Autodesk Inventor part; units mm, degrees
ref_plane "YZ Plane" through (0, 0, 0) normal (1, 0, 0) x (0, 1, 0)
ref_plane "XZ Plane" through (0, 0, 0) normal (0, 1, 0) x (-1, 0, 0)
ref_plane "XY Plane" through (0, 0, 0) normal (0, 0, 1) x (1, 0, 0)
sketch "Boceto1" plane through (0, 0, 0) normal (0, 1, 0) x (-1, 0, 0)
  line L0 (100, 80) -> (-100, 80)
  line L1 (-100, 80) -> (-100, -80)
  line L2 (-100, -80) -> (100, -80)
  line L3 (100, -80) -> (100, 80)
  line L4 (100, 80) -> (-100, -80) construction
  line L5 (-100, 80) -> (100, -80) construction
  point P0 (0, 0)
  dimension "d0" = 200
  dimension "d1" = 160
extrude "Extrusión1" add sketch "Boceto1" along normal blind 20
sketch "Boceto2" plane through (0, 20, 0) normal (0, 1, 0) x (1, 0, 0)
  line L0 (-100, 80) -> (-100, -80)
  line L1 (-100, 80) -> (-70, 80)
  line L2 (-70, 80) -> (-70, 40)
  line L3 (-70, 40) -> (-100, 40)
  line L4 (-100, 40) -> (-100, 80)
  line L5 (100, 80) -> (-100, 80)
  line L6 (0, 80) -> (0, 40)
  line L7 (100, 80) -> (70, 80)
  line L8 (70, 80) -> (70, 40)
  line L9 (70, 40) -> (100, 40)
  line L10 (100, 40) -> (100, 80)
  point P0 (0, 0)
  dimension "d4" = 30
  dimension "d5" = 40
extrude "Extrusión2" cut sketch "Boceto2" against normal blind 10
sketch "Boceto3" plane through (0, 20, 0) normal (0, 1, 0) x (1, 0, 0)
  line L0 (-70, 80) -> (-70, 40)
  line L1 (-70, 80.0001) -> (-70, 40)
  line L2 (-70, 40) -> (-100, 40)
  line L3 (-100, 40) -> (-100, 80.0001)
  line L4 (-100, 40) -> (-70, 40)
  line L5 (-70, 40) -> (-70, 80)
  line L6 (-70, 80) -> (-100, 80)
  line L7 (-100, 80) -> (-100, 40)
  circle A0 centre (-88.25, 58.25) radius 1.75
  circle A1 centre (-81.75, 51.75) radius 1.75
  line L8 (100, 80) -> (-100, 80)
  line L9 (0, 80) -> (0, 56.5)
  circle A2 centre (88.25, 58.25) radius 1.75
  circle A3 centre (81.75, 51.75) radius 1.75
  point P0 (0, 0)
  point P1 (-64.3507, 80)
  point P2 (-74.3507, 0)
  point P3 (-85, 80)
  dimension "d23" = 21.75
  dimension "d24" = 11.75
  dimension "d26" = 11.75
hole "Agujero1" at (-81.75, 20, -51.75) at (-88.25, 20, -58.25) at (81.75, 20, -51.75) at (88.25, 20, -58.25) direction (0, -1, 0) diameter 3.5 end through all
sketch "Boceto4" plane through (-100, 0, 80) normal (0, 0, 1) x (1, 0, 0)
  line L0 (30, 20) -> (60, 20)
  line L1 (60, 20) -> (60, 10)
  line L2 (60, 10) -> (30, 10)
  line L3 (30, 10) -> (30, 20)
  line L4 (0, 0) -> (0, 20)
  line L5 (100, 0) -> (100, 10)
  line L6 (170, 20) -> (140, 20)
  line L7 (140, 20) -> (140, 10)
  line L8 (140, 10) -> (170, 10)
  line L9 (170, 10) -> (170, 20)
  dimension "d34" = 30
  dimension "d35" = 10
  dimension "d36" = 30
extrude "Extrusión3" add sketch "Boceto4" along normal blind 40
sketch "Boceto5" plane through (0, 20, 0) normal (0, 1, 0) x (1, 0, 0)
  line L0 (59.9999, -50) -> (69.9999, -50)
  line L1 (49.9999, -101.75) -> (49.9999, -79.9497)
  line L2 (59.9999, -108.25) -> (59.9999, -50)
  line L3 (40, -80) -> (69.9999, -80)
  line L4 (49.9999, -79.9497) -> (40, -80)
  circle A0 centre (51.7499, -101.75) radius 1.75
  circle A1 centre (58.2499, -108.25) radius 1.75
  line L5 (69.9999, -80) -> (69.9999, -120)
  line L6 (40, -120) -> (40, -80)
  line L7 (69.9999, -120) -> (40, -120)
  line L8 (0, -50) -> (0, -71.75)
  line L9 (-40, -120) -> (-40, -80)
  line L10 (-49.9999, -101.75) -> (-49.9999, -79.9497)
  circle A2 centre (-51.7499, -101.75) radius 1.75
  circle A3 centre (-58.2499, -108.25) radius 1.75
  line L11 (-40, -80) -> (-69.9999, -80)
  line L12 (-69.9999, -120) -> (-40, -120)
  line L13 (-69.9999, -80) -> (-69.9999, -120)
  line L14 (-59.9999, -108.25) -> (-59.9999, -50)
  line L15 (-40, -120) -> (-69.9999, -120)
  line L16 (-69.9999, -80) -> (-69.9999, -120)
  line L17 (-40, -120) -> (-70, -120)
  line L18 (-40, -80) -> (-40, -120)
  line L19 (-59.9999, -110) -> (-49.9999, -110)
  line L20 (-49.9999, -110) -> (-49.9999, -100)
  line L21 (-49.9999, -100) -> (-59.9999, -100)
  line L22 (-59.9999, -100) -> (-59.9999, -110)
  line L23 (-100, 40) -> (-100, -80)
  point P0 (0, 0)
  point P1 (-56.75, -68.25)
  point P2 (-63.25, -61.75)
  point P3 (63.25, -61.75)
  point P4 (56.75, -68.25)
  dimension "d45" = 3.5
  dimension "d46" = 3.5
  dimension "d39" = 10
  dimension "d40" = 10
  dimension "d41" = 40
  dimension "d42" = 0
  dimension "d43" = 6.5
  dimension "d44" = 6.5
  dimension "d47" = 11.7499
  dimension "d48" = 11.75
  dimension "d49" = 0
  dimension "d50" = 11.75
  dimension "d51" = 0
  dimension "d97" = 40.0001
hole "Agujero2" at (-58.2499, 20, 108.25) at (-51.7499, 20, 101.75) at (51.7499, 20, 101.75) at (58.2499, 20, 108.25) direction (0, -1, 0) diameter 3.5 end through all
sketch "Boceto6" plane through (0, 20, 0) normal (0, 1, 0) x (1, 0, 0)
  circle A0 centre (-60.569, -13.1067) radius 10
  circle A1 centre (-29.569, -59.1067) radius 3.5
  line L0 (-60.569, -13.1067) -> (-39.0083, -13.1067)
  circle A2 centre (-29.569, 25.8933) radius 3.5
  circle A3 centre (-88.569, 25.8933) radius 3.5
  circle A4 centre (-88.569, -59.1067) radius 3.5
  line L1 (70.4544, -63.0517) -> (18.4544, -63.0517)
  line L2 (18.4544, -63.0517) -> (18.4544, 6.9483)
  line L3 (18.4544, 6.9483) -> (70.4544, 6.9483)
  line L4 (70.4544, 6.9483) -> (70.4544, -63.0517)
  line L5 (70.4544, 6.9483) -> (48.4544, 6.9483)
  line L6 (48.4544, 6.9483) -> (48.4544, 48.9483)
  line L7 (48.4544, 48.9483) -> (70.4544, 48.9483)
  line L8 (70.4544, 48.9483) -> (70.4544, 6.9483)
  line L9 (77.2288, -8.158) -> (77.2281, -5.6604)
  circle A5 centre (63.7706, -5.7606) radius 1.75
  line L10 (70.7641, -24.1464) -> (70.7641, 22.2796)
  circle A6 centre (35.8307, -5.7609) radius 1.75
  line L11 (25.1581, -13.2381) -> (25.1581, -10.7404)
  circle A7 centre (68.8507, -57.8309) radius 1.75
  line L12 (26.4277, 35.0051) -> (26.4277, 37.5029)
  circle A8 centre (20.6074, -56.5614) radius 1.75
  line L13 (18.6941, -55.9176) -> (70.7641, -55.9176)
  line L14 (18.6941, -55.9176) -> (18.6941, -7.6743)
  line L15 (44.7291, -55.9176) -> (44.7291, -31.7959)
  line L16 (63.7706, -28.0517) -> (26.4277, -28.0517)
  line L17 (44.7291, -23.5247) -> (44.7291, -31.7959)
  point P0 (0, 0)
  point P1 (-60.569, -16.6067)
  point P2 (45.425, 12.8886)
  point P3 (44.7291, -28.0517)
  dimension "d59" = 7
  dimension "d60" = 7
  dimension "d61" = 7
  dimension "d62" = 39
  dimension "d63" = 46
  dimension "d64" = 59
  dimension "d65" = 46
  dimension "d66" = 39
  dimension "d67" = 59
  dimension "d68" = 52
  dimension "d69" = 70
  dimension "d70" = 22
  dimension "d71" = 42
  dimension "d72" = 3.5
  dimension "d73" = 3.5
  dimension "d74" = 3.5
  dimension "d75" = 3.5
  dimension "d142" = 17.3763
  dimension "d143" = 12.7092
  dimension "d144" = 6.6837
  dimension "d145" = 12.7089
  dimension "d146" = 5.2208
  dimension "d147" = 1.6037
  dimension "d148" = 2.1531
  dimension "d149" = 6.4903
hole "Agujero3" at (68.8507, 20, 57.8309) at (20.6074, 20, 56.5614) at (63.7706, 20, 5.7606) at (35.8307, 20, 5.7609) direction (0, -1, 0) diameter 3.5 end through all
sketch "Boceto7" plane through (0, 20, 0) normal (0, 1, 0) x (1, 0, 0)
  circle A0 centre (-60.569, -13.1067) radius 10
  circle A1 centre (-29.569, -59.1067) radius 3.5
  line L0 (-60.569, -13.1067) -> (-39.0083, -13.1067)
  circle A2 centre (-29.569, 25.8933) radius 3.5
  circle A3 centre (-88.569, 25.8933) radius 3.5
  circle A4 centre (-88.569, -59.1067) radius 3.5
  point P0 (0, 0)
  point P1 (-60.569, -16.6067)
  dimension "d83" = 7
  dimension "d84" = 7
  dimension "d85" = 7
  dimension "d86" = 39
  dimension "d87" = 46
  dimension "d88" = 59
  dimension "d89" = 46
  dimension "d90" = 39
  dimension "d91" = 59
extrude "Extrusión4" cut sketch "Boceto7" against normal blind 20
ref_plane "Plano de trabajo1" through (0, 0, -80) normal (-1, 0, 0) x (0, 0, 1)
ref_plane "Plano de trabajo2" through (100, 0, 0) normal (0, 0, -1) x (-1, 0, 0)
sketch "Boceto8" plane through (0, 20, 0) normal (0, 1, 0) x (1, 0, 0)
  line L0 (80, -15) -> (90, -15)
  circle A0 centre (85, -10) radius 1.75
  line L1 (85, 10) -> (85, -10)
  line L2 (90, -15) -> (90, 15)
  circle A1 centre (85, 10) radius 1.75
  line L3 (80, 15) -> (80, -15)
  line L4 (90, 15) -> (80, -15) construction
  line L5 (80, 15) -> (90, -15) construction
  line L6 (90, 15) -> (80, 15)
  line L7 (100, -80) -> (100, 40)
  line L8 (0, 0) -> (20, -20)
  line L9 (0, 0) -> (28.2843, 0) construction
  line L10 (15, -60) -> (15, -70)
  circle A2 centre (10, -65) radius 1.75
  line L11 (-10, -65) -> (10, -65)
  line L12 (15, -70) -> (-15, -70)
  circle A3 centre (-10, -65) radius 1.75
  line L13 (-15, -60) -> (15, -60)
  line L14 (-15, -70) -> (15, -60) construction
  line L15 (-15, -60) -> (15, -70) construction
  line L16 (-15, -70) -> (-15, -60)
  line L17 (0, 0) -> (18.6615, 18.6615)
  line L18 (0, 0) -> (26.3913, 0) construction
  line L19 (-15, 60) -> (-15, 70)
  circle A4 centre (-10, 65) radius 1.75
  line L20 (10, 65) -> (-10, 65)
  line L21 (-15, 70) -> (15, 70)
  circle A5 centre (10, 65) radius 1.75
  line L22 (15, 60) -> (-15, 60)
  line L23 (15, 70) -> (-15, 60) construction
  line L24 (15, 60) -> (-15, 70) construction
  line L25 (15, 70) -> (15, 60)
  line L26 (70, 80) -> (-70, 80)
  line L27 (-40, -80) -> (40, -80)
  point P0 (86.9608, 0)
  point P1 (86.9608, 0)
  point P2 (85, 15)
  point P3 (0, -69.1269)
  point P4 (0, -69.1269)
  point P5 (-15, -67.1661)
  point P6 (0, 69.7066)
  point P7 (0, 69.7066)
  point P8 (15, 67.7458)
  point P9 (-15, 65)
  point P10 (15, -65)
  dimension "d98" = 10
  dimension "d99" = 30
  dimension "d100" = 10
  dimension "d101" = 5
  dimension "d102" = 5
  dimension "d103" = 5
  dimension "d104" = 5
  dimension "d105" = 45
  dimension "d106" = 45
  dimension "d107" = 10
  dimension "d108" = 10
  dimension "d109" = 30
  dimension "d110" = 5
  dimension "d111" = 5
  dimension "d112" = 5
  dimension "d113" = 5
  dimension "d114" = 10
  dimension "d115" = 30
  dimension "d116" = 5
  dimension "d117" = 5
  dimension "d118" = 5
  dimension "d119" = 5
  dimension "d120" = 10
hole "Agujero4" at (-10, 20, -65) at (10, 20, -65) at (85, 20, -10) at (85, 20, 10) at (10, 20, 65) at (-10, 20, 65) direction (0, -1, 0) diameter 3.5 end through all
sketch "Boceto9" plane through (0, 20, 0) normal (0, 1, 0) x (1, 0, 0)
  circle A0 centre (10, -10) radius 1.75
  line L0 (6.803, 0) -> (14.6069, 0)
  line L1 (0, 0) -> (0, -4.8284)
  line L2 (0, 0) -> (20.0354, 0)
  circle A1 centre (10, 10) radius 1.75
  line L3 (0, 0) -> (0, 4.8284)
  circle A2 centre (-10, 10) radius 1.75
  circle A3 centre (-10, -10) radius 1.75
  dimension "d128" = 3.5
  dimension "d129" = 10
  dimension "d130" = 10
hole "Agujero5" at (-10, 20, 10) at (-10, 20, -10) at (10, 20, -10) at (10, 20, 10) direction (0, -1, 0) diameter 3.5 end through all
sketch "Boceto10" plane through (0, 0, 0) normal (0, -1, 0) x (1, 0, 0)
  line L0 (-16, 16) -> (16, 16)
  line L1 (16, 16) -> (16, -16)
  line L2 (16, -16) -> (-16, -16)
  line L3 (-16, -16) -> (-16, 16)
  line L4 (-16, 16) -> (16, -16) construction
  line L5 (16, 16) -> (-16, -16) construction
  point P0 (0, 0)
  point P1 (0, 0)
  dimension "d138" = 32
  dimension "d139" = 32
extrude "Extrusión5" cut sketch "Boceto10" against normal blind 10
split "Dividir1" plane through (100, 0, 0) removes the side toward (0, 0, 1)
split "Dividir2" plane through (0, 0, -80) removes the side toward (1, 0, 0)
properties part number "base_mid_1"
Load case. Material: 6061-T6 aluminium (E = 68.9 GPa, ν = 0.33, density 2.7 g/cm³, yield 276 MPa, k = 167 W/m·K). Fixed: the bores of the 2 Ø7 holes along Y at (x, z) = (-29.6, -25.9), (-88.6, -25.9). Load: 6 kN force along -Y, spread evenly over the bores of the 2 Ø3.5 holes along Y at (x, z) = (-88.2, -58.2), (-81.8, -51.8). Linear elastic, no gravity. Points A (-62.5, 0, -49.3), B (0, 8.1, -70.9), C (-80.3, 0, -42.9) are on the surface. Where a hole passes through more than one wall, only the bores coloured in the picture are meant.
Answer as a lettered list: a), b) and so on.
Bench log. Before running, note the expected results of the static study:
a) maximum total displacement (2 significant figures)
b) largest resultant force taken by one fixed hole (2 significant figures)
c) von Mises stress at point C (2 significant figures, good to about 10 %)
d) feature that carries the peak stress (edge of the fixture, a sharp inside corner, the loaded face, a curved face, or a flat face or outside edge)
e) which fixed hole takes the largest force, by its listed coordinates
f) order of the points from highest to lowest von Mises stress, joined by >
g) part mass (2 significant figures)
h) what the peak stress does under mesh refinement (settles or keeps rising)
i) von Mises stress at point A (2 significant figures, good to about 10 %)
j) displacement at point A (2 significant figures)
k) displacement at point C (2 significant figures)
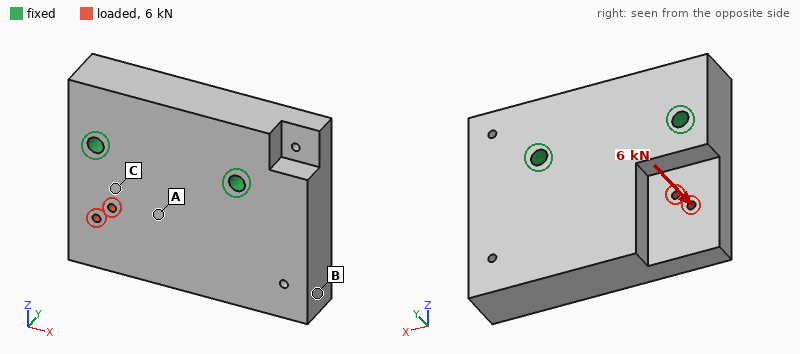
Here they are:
a) 0.14 mm
b) 5.4 kN
c) 50 MPa
d) a sharp inside corner
e) (-88.6, -25.9)
f) C > A > B
g) 390 g
h) keeps rising
i) 26 MPa
j) 0.030 mm
k) 0.029 mm
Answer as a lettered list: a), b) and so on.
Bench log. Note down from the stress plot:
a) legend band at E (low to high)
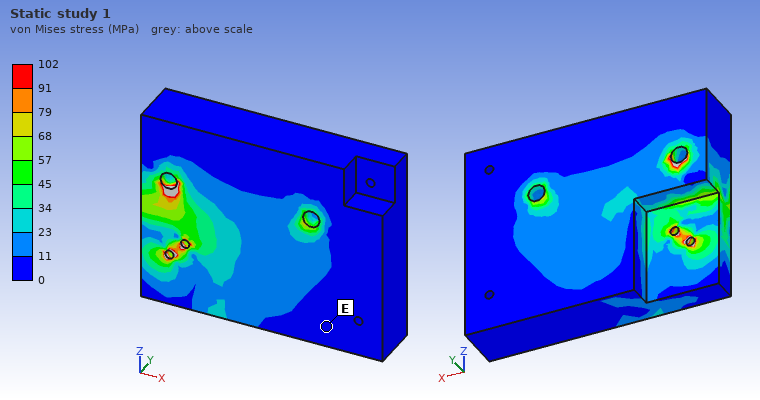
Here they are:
a) 0 to 11 MPa
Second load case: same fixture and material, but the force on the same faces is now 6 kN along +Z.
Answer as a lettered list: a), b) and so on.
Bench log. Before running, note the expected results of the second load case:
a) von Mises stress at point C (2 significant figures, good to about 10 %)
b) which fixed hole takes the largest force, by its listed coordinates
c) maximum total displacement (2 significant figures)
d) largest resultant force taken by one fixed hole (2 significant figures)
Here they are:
a) 19 MPa
b) (-88.6, -25.9)
c) 14 µm
d) 5.6 kN
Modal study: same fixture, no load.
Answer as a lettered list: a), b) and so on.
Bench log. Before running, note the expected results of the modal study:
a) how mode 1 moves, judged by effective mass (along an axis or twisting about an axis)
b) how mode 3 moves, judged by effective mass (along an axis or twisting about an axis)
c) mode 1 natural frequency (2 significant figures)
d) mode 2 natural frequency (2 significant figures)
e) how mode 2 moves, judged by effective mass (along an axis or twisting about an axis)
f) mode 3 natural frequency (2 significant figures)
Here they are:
a) along Y
b) along X
c) 4000 Hz
d) 6300 Hz
e) twisting about Z
f) 8900 Hz
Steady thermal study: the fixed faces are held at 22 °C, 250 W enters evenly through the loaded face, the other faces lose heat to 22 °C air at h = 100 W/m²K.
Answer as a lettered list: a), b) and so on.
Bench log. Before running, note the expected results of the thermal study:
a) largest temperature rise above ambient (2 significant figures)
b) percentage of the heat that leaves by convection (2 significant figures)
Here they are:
a) 84 K
b) 14 %
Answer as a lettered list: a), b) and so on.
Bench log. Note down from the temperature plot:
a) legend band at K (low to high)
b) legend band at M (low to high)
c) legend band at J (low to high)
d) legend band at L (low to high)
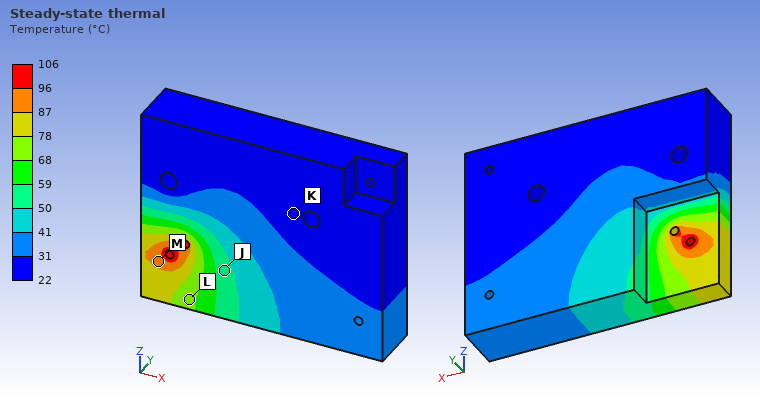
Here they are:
a) 22 to 31 °C
b) 87 to 96 °C
c) 50 to 59 °C
d) 68 to 78 °C
